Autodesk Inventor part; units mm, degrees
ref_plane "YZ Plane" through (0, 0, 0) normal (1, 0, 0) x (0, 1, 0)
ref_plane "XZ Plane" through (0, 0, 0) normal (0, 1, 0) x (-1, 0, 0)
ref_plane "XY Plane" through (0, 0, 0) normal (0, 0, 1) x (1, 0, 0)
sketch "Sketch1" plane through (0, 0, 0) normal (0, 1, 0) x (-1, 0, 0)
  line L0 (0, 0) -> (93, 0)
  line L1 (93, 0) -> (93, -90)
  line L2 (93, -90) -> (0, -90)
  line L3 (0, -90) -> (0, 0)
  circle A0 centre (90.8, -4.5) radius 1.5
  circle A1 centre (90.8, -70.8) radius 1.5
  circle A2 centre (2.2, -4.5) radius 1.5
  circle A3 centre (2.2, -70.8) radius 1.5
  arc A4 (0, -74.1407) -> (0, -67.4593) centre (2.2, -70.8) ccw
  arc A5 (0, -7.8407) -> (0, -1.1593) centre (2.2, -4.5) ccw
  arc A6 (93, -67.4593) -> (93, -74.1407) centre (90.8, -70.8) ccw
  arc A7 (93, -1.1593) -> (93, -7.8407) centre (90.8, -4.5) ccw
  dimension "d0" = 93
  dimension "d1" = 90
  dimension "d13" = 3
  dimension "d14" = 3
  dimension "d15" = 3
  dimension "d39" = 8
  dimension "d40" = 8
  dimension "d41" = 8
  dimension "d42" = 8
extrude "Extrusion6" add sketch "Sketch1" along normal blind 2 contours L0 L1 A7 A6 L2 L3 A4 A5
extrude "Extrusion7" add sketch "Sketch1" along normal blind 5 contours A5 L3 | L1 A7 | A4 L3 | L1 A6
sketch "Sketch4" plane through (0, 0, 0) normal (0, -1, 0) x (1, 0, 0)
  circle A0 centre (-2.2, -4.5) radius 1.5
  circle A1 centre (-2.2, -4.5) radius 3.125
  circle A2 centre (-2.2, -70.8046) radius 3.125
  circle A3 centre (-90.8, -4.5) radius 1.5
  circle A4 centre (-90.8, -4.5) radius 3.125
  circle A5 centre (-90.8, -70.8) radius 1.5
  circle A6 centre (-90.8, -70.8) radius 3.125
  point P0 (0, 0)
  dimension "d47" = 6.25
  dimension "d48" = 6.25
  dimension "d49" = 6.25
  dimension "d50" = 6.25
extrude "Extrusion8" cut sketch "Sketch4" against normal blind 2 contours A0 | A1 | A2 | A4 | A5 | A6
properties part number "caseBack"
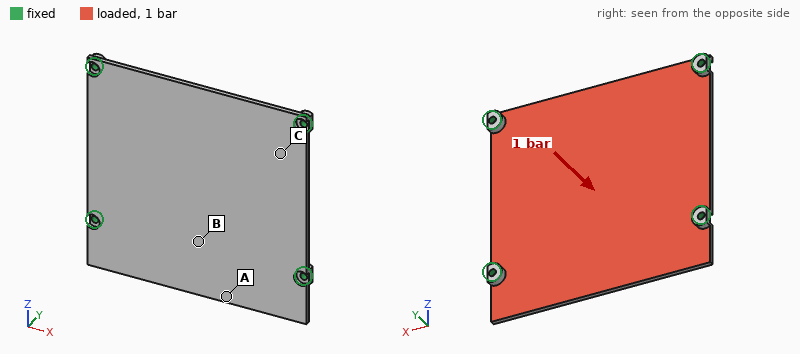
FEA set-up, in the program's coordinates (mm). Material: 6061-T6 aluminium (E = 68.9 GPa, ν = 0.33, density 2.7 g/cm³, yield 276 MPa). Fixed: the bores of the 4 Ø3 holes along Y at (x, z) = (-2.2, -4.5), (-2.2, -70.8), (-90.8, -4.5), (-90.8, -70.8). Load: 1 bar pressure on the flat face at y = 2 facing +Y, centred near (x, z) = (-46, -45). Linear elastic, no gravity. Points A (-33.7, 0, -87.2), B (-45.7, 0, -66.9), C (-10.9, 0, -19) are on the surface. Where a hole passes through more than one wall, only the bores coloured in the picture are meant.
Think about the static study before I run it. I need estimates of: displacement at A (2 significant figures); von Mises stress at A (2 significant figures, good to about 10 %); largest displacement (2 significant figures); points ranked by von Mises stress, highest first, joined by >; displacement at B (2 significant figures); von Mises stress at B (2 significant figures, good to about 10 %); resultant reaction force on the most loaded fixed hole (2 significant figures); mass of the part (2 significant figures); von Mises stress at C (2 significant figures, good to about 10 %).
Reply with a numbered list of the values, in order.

1. 0.42 mm
2. 50 MPa
3. 0.59 mm
4. B > A > C
5. 0.51 mm
6. 65 MPa
7. 640 N
8. 46 g
9. 29 MPa
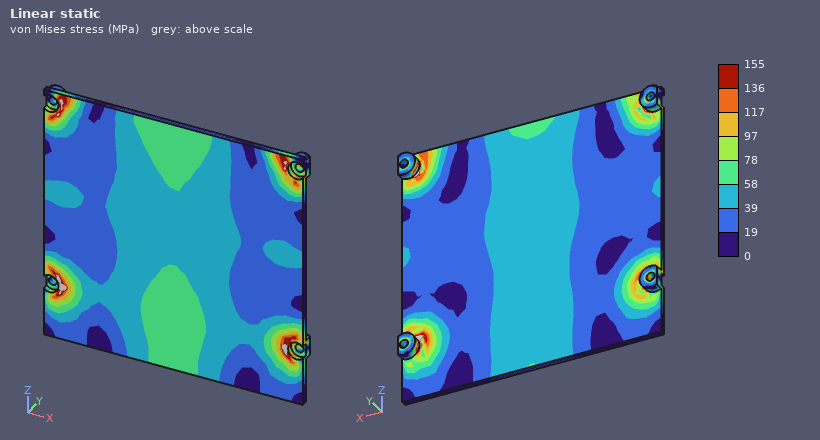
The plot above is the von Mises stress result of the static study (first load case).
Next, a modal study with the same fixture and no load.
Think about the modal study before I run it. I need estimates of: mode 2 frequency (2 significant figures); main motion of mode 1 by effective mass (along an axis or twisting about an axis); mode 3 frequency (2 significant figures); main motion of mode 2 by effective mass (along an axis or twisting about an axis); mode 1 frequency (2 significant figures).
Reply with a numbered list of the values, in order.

1. 1400 Hz
2. along Y
3. 2100 Hz
4. twisting about X
5. 1100 Hz
